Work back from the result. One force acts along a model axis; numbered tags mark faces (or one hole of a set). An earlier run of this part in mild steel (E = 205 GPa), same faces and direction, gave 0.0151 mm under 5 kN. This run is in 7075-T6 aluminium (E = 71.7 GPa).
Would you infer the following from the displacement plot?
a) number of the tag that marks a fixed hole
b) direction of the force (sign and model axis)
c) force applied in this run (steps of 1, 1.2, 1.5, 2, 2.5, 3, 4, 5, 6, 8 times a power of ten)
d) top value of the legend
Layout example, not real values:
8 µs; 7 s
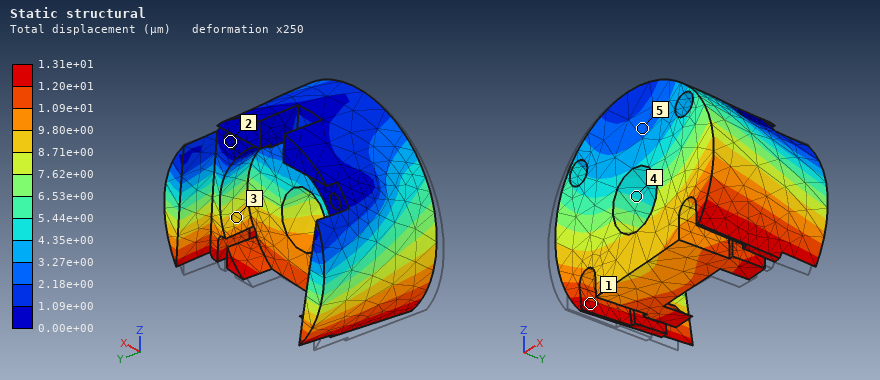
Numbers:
2; +X; 1.5 kN; 1.31e+01 µm
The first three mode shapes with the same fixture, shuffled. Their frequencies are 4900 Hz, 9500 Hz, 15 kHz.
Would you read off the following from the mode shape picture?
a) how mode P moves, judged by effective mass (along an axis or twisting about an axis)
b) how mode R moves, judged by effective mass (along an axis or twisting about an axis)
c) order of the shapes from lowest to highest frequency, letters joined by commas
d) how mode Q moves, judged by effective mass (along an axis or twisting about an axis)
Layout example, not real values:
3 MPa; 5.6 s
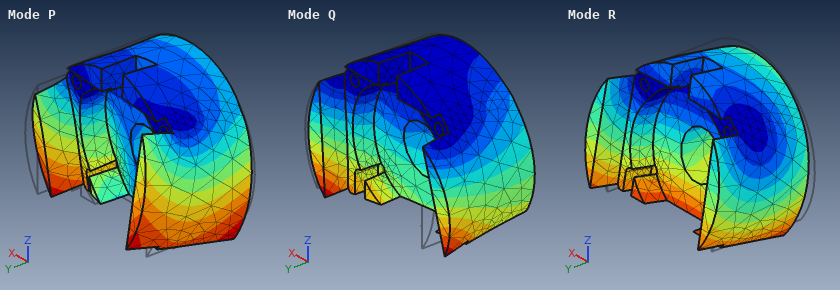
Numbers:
along X; along Y; R, Q, P; along X
